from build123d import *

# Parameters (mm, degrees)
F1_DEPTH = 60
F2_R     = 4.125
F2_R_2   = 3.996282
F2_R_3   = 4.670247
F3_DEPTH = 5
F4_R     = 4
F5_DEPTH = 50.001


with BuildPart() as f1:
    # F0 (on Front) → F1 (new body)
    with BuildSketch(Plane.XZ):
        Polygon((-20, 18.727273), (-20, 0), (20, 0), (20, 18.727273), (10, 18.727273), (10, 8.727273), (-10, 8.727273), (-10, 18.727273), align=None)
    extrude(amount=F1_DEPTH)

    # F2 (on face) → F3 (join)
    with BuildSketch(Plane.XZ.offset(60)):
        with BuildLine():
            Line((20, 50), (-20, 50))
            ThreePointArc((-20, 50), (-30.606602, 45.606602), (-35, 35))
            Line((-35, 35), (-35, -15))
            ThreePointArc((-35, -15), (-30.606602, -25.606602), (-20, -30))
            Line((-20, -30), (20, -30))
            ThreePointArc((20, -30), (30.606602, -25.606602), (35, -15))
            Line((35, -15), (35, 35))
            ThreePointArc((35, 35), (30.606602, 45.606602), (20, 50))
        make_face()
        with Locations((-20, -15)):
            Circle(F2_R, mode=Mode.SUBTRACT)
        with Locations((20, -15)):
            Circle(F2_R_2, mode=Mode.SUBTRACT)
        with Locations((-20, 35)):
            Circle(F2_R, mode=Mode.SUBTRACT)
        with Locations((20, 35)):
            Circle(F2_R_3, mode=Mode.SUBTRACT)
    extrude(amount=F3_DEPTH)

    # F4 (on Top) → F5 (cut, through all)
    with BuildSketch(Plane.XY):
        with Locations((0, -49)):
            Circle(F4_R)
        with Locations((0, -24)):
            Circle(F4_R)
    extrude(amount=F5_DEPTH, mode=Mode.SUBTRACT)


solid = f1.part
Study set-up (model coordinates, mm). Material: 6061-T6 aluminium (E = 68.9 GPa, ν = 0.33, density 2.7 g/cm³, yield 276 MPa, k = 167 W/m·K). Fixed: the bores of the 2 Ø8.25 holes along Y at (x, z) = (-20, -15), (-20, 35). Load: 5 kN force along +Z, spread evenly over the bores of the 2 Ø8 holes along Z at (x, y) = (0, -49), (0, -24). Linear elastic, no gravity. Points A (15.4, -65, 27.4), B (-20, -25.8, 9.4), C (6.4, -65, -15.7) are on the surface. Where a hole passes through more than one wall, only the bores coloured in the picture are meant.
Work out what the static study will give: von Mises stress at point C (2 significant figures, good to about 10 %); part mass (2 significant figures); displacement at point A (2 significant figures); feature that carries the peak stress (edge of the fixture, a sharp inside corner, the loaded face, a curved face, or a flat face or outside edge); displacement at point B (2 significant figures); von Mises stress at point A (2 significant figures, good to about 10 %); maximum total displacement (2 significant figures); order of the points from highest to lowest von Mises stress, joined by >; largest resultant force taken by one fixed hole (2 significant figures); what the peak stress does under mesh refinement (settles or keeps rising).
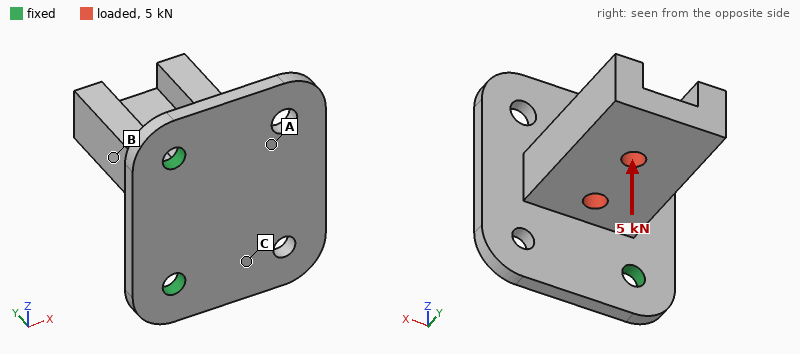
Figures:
44 MPa
160 g
0.15 mm
edge of the fixture
0.27 mm
72 MPa
0.59 mm
A > C > B
4.6 kN
keeps rising
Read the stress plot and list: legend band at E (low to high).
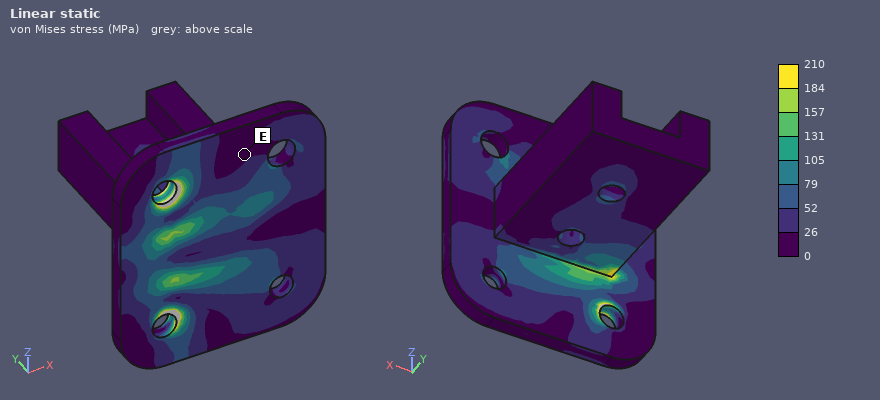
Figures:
0 to 26 MPa
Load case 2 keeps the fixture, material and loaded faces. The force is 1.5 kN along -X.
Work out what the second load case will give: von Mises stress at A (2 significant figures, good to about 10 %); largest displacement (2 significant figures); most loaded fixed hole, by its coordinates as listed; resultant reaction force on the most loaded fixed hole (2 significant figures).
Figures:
16 MPa
0.51 mm
(-20, -15)
930 N
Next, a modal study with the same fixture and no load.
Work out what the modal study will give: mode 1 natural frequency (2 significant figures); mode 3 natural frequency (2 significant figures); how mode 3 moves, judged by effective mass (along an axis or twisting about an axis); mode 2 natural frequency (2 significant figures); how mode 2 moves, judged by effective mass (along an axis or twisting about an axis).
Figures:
840 Hz
4000 Hz
along Y
1700 Hz
along Z
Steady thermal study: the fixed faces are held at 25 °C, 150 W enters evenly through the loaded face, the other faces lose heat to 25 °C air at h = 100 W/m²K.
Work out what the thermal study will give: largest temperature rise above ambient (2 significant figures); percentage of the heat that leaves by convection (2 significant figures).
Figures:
68 K
44 %
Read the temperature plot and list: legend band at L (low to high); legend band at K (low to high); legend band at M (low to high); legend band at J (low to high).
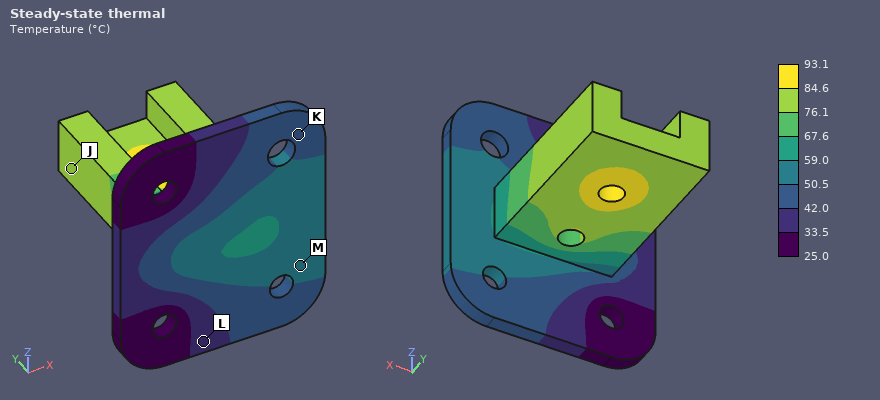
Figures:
33.5 to 42.0 °C
42.0 to 50.5 °C
50.5 to 59.0 °C
76.1 to 84.6 °C
